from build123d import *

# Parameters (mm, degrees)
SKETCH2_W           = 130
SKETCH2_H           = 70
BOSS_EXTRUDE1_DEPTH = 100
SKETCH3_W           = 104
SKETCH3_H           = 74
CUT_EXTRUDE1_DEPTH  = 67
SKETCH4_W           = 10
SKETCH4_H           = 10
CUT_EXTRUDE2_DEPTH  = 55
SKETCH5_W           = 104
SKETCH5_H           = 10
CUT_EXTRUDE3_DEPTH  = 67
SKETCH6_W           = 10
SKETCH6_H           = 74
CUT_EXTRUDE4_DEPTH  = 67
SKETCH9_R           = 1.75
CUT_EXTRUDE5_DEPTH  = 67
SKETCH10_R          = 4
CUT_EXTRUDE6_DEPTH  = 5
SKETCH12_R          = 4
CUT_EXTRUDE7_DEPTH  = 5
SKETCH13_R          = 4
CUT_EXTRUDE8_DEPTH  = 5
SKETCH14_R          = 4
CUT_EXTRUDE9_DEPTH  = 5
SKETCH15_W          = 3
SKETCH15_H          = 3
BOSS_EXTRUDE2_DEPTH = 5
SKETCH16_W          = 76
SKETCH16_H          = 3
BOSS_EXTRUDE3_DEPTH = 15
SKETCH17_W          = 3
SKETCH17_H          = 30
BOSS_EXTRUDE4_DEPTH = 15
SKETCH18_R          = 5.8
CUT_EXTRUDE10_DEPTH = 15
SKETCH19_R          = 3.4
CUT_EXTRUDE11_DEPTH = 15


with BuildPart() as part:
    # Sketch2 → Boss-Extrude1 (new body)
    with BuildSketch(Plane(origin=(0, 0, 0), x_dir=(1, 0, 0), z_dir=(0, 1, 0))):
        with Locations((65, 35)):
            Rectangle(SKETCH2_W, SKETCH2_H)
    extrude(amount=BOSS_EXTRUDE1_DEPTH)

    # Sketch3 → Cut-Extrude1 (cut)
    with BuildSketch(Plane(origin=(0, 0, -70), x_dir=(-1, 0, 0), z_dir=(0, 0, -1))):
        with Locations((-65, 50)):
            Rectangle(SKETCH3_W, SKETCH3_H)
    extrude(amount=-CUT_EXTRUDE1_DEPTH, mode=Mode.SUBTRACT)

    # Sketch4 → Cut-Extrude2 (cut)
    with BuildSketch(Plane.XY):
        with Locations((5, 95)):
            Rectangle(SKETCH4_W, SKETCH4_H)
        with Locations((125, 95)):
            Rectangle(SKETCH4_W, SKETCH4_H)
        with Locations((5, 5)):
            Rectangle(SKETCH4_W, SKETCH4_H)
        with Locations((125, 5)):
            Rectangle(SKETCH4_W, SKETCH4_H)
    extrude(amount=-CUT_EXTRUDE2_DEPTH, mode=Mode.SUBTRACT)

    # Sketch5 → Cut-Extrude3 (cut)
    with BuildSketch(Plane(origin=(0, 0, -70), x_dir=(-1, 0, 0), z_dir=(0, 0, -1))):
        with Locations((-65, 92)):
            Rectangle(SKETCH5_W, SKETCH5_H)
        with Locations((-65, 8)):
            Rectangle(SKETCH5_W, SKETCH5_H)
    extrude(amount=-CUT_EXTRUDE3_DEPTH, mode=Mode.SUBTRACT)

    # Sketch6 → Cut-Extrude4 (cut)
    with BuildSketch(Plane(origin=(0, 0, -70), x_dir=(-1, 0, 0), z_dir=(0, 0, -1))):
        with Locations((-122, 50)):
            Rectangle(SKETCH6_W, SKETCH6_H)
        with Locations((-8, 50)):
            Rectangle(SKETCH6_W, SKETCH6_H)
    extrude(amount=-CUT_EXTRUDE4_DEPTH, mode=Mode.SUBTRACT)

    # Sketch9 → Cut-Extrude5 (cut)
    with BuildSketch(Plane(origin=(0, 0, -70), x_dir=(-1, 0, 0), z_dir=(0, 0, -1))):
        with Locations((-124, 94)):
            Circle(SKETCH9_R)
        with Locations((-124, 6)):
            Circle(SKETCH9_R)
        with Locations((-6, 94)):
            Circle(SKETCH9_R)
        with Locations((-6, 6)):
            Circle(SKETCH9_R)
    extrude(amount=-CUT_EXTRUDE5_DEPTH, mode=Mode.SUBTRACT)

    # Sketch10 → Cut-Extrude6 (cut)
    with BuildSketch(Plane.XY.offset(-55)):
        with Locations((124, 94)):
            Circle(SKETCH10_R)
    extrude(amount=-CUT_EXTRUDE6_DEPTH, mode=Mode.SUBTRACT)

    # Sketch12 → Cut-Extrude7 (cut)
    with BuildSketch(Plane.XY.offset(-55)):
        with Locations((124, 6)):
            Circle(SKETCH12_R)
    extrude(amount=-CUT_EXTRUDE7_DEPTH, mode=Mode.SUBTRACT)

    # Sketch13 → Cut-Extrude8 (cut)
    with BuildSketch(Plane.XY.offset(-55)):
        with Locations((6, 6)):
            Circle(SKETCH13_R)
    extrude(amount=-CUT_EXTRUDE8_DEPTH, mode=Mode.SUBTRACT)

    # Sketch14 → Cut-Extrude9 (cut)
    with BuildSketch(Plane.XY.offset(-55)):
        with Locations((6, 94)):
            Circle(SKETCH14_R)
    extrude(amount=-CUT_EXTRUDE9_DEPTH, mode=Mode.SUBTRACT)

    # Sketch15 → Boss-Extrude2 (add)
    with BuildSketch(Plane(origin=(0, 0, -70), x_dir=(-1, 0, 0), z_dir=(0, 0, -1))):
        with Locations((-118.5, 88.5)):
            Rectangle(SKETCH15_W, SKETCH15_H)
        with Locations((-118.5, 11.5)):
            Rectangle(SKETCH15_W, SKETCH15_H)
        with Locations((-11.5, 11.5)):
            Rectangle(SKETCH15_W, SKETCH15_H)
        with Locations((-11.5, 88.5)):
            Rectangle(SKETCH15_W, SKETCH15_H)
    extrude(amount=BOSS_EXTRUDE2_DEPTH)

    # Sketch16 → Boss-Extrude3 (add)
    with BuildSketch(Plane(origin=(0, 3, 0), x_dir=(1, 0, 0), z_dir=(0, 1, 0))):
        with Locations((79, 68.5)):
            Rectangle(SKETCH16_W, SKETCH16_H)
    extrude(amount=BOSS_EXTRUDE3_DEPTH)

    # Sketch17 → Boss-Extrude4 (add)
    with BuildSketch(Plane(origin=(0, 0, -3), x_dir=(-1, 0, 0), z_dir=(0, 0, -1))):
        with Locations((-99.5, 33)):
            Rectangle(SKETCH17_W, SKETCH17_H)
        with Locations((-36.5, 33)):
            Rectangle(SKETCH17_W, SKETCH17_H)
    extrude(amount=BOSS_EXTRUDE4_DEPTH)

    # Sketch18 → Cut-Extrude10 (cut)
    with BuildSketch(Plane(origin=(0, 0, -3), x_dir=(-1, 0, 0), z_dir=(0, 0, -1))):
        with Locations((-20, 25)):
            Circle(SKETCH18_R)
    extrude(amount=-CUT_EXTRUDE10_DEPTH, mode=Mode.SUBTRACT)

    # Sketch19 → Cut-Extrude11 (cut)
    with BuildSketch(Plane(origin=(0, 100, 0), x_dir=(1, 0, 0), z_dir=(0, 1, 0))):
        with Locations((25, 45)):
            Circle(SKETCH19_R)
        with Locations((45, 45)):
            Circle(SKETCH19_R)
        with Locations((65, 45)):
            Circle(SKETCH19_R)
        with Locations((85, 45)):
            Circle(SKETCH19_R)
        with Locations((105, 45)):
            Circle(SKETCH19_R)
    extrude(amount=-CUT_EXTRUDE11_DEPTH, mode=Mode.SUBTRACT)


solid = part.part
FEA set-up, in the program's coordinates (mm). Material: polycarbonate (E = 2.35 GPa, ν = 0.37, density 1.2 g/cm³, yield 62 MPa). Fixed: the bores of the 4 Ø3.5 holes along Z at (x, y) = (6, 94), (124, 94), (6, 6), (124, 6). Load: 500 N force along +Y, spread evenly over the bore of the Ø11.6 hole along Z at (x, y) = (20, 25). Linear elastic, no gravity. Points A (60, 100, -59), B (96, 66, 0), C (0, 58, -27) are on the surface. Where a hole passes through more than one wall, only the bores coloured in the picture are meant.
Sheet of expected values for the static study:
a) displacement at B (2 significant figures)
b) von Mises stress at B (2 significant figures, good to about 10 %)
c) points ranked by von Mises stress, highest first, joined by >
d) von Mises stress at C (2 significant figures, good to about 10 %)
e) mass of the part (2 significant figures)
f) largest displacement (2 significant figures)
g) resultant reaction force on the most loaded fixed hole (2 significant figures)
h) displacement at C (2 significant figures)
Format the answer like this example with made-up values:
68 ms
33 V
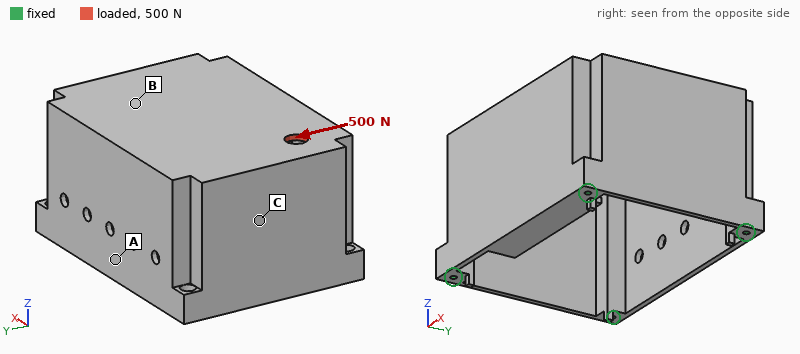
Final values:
0.11 mm
0.95 MPa
C > B > A
2.9 MPa
170 g
0.21 mm
280 N
0.093 mm
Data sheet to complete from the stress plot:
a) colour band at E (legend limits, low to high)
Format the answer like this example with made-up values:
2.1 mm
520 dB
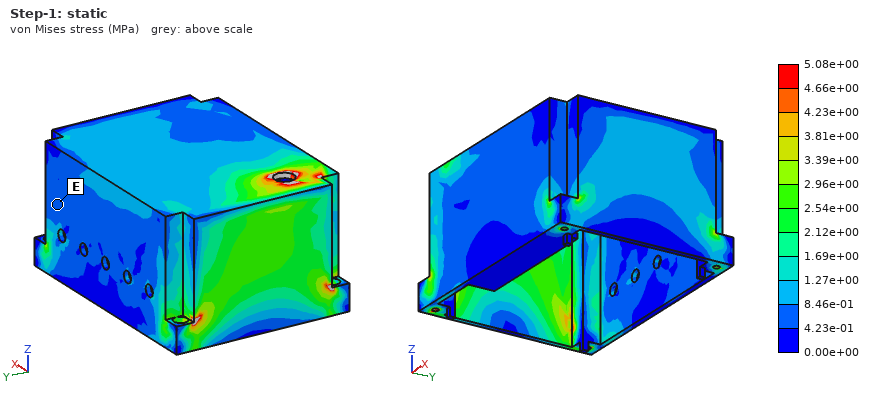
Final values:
4.23e-01 to 8.46e-01 MPa
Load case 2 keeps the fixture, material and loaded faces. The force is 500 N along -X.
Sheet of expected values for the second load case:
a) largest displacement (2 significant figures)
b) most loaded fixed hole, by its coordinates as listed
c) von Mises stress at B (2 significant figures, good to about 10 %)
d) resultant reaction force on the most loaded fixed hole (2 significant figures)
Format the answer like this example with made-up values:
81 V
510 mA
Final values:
0.18 mm
(124, 6)
0.83 MPa
230 N
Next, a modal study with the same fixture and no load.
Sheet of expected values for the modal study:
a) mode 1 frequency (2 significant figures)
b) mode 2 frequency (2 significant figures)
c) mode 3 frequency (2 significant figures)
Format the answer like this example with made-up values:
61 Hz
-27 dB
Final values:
430 Hz
510 Hz
620 Hz
